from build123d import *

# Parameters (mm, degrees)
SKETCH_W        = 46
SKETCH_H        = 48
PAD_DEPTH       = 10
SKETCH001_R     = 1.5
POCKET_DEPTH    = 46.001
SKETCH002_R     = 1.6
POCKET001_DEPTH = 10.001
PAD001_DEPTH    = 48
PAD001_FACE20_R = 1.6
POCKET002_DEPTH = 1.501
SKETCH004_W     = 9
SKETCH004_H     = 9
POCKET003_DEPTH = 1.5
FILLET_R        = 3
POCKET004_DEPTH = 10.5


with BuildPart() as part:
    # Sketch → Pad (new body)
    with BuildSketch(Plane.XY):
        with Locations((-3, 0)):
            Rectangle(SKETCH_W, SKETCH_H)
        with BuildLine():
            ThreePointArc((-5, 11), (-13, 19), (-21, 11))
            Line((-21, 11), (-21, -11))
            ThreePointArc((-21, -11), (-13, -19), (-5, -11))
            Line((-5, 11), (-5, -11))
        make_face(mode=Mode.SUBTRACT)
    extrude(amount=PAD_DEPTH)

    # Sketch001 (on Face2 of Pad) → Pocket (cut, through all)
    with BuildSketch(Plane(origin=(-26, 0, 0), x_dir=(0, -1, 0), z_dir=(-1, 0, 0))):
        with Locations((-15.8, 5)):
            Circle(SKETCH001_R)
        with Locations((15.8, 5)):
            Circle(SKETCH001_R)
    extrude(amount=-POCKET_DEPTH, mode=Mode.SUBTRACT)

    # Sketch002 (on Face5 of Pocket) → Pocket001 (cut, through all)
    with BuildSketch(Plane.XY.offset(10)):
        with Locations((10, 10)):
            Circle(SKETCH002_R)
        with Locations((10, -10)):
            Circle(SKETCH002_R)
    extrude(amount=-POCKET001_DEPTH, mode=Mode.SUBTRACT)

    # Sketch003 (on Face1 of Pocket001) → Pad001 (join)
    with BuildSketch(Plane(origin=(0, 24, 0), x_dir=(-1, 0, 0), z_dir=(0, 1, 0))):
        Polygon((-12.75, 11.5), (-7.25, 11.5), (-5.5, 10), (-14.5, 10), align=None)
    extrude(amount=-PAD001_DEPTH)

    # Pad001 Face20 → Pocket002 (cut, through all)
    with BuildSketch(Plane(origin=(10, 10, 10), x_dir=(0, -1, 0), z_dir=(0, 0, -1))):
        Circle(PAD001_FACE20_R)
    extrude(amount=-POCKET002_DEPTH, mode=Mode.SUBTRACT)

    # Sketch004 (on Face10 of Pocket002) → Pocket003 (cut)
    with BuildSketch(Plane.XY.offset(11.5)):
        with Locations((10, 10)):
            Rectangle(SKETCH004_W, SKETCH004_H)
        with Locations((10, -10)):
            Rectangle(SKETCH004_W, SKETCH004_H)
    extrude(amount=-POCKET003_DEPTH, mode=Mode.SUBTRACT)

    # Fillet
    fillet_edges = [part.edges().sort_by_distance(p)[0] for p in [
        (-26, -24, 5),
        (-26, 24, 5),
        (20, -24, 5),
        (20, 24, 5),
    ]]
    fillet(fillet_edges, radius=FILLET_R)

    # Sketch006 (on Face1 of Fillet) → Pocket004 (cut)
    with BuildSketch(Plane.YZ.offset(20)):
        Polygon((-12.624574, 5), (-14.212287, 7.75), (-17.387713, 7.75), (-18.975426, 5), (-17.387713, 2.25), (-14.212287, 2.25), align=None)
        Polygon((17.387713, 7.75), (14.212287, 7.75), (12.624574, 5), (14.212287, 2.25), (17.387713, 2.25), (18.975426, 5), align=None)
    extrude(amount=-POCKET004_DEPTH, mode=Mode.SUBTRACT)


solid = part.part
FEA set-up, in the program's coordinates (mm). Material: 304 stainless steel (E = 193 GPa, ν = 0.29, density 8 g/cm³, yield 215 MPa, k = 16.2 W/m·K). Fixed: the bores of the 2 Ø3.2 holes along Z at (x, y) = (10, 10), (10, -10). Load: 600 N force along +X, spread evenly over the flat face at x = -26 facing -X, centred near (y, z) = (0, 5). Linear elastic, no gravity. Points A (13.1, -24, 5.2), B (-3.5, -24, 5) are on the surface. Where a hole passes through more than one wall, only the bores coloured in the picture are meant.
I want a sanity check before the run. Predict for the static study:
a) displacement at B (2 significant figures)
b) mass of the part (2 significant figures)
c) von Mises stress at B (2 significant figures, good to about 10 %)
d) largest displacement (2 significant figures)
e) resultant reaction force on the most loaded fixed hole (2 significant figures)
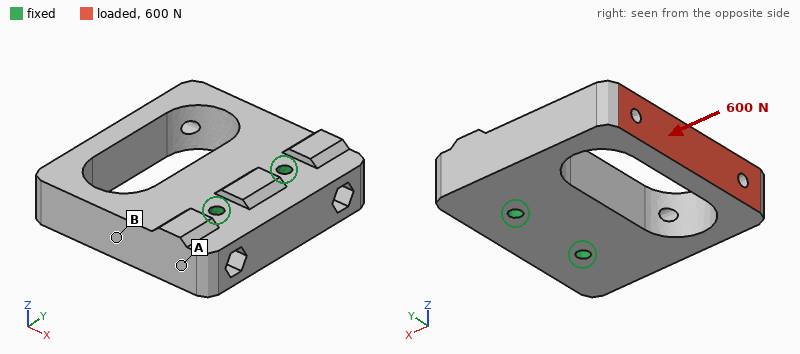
1.3 µm
130 g
9.4 MPa
8.3 µm
320 N
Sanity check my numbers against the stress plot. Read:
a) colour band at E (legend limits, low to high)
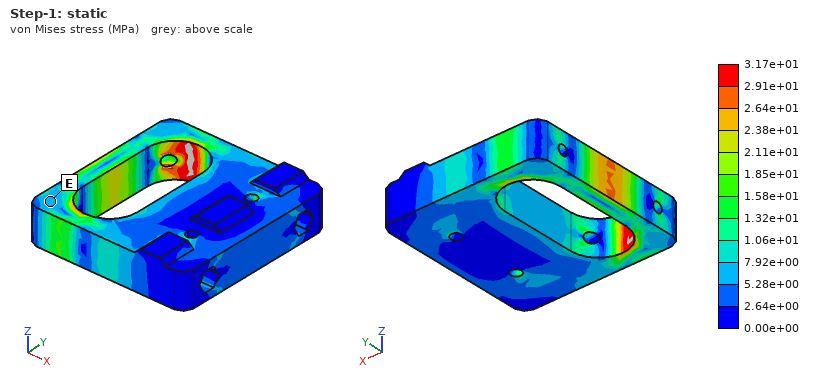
5.28e+00 to 7.92e+00 MPa
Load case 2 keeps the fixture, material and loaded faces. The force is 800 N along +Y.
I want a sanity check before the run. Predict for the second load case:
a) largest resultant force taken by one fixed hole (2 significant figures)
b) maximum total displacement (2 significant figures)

1.3 kN
20 µm
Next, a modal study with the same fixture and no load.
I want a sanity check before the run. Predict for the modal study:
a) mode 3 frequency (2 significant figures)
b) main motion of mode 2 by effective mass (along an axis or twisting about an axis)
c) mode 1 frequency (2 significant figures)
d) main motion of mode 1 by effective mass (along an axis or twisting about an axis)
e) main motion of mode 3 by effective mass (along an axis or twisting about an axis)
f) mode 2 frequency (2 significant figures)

7600 Hz
along Y
4600 Hz
along Z
twisting about X
6900 Hz
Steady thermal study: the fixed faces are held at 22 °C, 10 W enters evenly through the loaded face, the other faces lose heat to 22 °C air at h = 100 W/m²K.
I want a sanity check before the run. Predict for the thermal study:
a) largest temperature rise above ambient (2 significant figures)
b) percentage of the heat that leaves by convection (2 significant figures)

69 K
85 %
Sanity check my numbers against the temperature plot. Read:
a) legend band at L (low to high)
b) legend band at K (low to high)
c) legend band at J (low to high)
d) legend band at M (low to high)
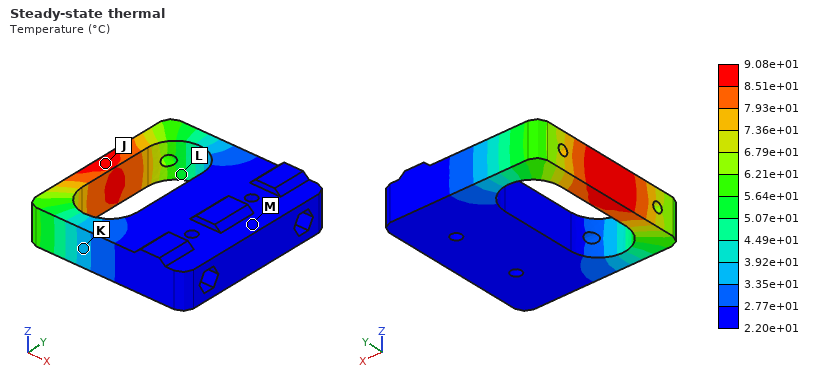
5.07e+01 to 5.64e+01 °C
3.35e+01 to 3.92e+01 °C
8.51e+01 to 9.08e+01 °C
2.20e+01 to 2.77e+01 °C
